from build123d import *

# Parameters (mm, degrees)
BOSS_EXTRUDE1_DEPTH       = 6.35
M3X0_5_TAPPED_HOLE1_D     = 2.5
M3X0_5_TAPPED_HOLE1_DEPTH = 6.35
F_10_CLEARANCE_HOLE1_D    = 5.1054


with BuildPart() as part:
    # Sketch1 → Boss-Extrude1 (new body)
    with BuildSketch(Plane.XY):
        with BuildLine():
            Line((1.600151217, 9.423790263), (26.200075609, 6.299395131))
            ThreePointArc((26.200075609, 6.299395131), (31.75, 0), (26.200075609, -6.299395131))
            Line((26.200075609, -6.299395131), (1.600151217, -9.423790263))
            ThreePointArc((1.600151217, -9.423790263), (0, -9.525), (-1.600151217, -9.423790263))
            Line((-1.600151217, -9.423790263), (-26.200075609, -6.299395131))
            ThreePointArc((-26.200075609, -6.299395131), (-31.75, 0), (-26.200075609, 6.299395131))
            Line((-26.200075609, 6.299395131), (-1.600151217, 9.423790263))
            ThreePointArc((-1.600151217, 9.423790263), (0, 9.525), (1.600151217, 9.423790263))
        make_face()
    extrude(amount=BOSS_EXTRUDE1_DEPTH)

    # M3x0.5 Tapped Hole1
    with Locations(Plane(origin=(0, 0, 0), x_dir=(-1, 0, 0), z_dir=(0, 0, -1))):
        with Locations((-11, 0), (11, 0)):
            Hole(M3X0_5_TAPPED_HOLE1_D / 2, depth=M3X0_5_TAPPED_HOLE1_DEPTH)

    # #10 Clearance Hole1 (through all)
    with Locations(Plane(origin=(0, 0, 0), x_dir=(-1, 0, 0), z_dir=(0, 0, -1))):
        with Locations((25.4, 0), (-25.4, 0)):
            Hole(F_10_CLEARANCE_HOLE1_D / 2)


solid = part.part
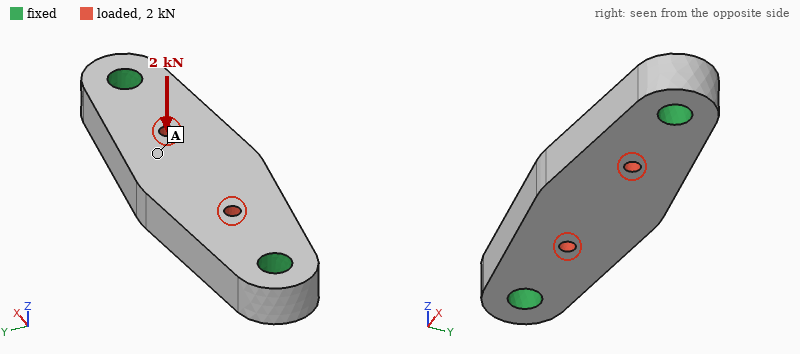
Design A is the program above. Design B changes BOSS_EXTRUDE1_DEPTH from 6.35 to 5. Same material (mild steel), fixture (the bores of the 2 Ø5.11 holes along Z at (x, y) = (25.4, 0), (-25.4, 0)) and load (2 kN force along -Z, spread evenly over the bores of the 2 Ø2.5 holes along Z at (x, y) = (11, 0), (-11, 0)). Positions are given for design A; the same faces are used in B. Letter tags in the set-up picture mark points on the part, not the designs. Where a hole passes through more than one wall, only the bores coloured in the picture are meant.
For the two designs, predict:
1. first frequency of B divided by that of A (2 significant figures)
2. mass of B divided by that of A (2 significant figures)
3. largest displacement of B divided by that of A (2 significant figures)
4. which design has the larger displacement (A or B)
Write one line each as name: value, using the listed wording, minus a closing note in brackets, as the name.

first frequency of B divided by that of A: 0.83
mass of B divided by that of A: 0.79
largest displacement of B divided by that of A: 1.9
which design has the larger displacement: B
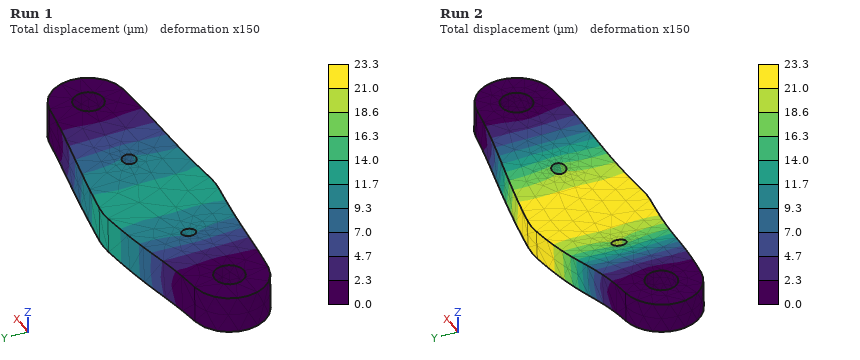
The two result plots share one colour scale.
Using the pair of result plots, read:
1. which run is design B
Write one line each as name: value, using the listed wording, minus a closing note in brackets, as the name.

which run is design B: Run 2
